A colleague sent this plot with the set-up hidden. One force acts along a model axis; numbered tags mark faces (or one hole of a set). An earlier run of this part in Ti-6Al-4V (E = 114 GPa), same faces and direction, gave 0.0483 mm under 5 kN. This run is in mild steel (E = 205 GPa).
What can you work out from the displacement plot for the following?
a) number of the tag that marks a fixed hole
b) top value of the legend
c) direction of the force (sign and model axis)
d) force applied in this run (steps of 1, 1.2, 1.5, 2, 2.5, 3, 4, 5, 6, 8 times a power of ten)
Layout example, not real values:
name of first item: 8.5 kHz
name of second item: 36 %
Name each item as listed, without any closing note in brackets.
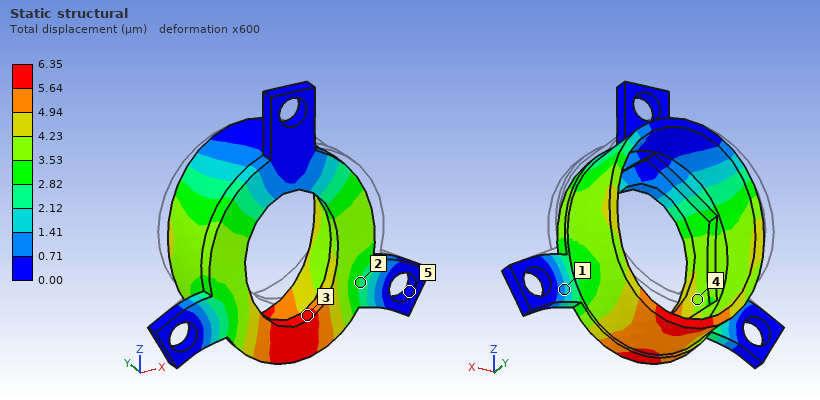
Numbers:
number of the tag that marks a fixed hole: 5
top value of the legend: 6.35 µm
direction of the force: -Z
force applied in this run: 1.2 kN
